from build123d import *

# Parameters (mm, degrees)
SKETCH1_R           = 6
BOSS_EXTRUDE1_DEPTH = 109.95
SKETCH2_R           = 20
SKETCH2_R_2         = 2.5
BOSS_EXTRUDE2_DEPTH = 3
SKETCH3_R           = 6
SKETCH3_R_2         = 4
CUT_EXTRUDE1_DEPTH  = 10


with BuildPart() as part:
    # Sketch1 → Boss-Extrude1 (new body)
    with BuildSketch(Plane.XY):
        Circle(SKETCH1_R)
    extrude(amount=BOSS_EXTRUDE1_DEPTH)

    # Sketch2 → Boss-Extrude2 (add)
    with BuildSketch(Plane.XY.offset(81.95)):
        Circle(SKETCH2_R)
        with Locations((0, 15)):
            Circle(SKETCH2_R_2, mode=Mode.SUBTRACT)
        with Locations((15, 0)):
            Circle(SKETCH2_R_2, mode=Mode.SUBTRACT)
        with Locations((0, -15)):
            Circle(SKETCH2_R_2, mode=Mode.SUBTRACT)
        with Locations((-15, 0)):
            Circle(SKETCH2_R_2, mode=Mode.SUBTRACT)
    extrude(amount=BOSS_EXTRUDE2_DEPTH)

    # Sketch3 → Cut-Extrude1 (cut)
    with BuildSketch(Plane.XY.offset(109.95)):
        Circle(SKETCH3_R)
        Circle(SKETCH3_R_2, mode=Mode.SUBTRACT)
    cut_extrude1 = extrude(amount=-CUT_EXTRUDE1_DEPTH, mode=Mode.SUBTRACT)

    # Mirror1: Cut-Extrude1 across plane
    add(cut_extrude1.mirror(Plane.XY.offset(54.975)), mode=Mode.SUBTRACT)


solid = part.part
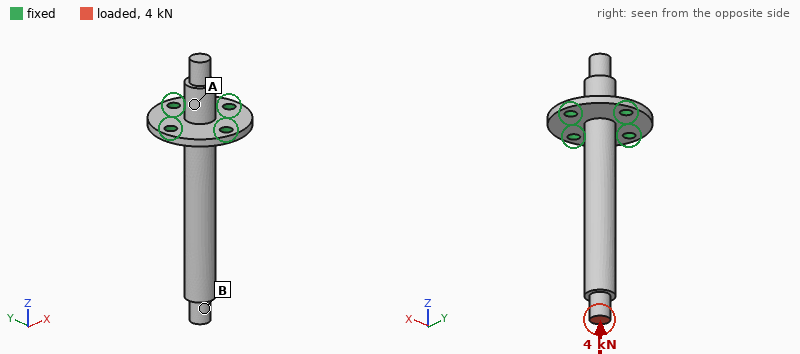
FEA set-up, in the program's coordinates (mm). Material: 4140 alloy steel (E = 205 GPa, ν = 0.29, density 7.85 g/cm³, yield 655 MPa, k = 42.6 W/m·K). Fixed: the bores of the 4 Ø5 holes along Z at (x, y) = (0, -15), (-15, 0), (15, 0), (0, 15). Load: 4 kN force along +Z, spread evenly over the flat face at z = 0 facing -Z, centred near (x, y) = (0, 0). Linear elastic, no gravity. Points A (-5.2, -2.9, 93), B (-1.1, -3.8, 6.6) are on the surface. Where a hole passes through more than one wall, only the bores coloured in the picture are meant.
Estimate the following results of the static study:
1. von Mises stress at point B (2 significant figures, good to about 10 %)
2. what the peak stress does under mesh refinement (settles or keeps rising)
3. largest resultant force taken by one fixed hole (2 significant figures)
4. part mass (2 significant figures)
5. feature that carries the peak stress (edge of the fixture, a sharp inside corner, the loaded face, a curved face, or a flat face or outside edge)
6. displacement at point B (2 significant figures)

78 MPa
keeps rising
1.0 kN
110 g
edge of the fixture
26 µm
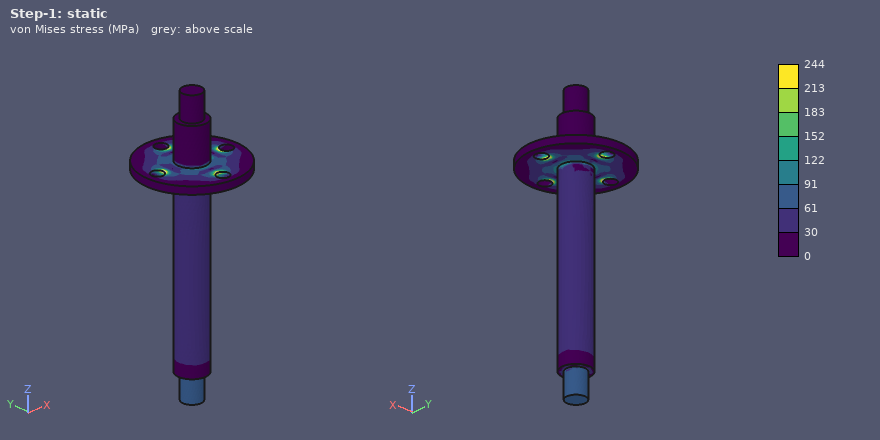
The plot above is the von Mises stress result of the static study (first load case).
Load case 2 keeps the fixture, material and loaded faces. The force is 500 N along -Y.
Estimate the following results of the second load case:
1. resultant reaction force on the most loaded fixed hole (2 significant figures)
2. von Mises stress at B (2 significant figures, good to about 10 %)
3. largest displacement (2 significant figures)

1.8 kN
62 MPa
0.66 mm
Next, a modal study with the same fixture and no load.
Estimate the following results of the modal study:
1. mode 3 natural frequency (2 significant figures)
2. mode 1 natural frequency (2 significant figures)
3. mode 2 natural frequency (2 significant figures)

6600 Hz
1100 Hz
1100 Hz
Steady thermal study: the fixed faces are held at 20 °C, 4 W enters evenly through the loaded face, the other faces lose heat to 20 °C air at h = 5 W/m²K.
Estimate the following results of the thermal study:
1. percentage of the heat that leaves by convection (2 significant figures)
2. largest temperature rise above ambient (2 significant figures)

14 %
79 K
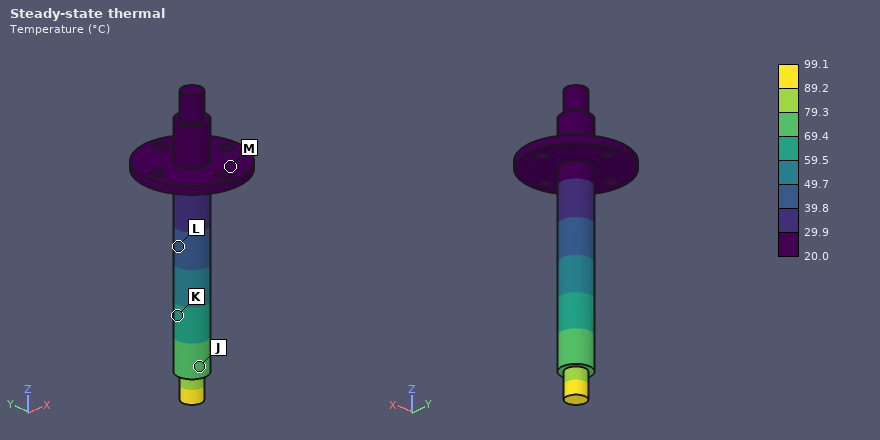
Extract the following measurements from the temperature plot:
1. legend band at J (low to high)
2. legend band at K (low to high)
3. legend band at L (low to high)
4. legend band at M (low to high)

69.4 to 79.3 °C
59.5 to 69.4 °C
39.8 to 49.7 °C
20.0 to 29.9 °C
